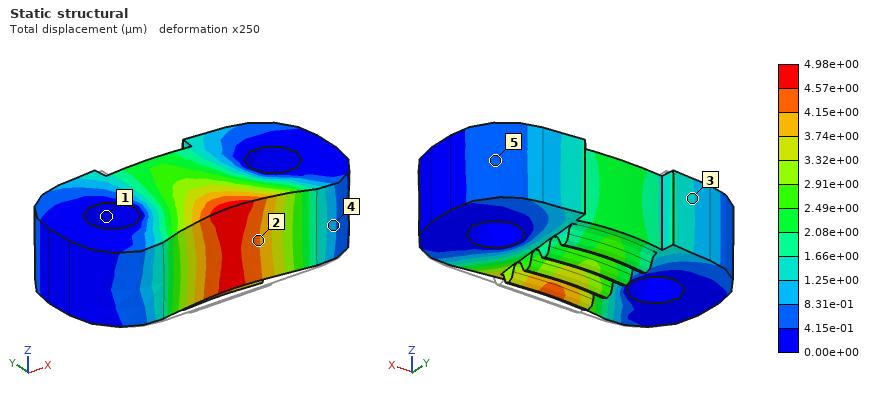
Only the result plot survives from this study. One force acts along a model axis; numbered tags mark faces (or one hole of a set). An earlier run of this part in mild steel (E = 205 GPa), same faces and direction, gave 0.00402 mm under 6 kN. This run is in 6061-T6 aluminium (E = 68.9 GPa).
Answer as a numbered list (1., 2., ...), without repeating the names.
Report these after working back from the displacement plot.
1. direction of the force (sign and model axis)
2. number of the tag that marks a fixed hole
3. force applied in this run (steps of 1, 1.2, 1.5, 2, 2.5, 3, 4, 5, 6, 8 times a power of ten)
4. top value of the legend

1. +Y
2. 1
3. 2.5 kN
4. 4.98e+00 µm
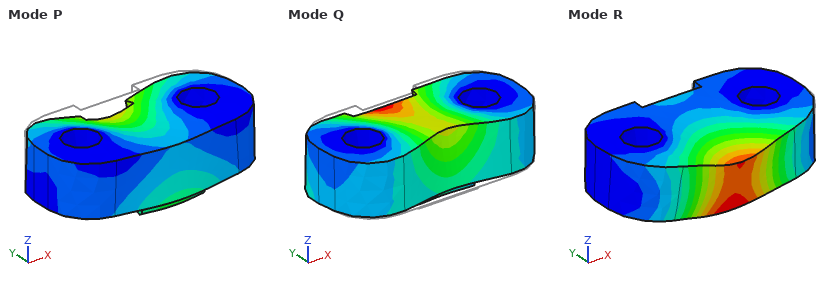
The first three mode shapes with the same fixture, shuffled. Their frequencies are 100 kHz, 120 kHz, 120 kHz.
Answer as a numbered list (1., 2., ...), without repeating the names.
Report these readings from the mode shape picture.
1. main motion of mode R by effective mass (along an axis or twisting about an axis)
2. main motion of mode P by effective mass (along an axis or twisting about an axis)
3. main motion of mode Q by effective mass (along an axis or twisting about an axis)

1. along Z
2. along Z
3. along Y
